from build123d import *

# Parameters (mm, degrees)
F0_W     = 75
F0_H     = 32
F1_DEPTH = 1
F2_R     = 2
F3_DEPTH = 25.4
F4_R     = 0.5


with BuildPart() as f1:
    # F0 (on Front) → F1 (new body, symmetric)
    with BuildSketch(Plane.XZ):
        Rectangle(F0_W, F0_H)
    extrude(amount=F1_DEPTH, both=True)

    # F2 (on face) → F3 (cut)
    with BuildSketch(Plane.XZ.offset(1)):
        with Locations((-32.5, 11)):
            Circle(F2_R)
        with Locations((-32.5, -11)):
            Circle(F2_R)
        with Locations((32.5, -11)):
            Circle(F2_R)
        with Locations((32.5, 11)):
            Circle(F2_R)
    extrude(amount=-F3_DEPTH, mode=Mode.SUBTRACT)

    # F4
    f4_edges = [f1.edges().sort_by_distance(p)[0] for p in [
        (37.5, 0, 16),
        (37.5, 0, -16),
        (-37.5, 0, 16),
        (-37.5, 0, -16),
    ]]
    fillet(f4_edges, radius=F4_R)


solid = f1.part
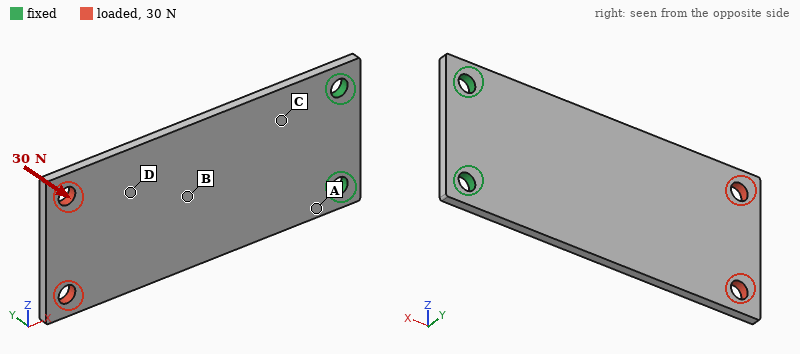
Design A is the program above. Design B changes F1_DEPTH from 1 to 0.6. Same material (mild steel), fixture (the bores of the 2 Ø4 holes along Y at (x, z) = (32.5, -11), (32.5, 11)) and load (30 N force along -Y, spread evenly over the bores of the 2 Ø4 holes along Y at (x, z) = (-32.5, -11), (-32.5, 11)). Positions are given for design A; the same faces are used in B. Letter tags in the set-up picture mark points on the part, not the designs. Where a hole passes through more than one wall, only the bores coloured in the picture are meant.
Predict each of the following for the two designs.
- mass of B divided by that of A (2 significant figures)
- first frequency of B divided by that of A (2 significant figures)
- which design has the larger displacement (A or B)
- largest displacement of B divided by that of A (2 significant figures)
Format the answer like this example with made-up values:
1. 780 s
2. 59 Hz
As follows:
1. 0.60
2. 0.60
3. B
4. 4.6
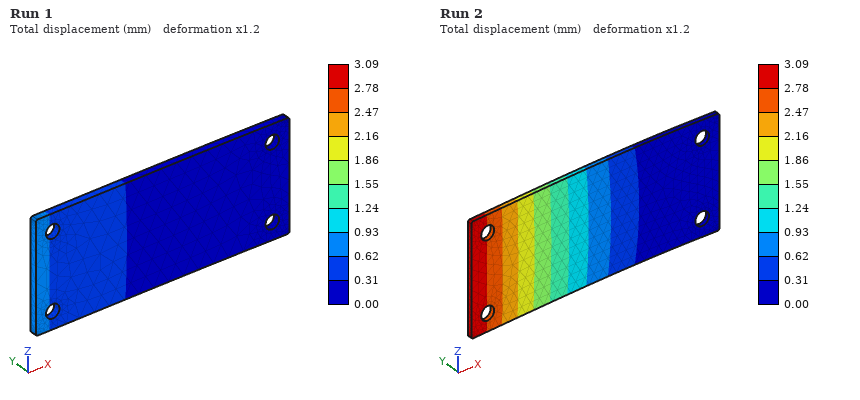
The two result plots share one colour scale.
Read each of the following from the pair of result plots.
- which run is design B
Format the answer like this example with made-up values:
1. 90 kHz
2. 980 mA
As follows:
1. Run 2
